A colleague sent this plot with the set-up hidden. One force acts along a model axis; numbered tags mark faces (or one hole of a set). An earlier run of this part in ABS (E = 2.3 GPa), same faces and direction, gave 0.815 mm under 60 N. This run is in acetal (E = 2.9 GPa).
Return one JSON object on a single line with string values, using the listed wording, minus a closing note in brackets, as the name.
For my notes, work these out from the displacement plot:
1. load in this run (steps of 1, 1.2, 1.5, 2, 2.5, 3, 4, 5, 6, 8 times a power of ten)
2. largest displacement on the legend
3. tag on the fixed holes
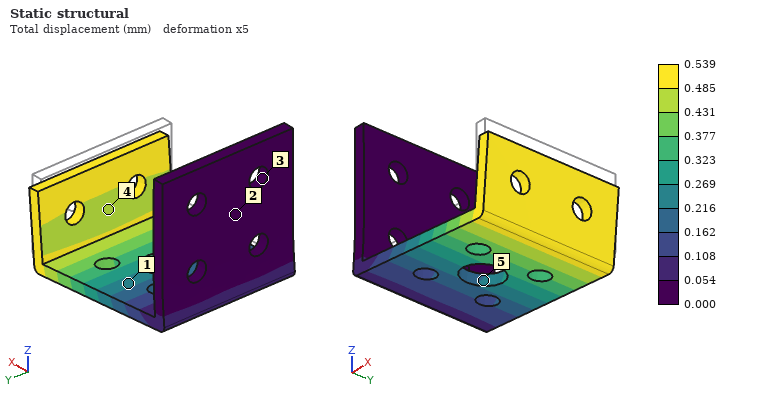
{"load in this run": "50 N", "largest displacement on the legend": "0.539 mm", "tag on the fixed holes": "3"}
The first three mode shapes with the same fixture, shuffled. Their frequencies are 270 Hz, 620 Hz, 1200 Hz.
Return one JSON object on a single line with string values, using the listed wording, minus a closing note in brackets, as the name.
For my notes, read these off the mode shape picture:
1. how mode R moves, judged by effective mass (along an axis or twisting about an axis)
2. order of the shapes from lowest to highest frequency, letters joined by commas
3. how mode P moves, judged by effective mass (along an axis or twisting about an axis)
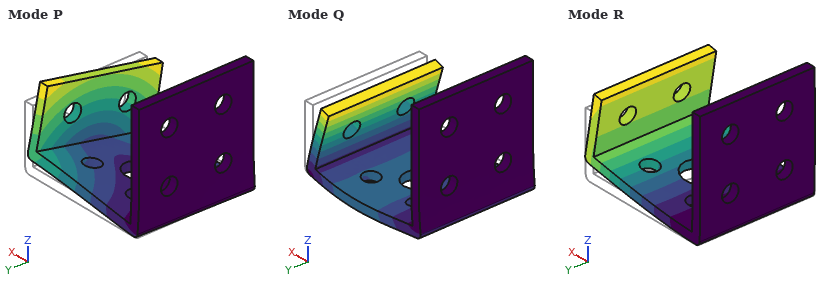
{"how mode R moves, judged by effective mass": "along Z", "order of the shapes from lowest to highest frequency, letters joined by commas": "R, P, Q", "how mode P moves, judged by effective mass": "along Y"}
